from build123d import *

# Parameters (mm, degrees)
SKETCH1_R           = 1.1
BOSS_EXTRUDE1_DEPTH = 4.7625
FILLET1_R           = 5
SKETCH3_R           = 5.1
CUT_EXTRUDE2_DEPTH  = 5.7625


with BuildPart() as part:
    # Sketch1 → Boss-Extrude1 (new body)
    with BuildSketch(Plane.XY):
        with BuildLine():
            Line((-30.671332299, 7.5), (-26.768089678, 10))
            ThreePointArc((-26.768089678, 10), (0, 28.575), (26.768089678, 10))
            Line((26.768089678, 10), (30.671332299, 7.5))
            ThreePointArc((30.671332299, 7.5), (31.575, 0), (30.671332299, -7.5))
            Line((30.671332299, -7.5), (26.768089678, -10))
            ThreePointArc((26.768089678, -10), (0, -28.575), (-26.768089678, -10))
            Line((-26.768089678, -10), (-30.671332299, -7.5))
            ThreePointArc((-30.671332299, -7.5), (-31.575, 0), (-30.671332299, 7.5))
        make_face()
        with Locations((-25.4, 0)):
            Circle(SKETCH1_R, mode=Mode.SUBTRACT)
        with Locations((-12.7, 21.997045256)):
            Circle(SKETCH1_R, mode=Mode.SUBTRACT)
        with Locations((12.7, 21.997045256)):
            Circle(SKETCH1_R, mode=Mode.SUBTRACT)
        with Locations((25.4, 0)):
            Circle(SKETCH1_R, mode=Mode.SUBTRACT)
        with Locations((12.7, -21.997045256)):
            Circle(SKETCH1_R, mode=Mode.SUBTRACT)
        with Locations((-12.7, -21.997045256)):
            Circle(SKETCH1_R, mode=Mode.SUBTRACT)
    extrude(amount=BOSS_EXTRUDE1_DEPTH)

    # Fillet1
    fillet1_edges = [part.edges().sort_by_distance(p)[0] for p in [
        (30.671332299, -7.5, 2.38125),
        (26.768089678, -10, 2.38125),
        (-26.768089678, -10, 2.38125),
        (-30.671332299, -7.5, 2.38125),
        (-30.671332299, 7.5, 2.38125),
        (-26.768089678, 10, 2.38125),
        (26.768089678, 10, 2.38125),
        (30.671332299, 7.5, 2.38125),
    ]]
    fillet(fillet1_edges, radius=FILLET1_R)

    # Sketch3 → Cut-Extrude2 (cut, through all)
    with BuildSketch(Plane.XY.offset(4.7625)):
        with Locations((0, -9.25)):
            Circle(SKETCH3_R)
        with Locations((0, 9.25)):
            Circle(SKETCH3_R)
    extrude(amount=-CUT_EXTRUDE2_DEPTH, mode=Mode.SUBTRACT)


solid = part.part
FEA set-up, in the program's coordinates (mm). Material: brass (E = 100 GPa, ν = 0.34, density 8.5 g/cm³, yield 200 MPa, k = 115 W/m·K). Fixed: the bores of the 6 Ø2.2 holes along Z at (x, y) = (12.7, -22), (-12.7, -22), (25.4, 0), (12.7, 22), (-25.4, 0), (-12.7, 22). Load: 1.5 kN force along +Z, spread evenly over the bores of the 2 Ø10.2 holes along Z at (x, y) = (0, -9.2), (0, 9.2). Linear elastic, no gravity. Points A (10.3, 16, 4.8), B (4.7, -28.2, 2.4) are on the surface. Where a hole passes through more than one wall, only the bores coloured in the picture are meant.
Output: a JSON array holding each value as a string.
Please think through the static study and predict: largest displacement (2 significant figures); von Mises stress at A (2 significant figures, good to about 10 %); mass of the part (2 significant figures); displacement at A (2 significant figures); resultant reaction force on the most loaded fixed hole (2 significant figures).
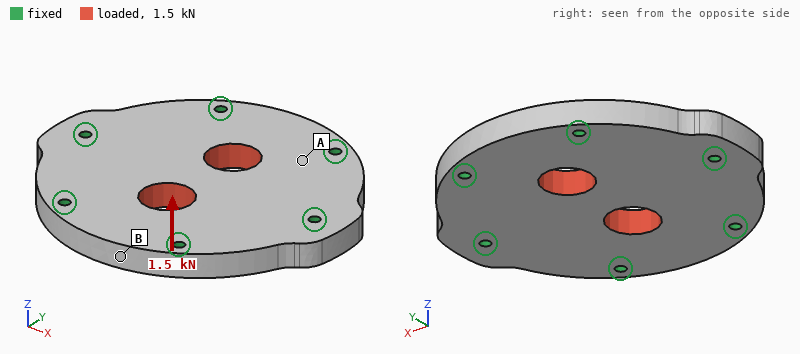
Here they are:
["26 µm", "22 MPa", "100 g", "6.7 µm", "290 N"]
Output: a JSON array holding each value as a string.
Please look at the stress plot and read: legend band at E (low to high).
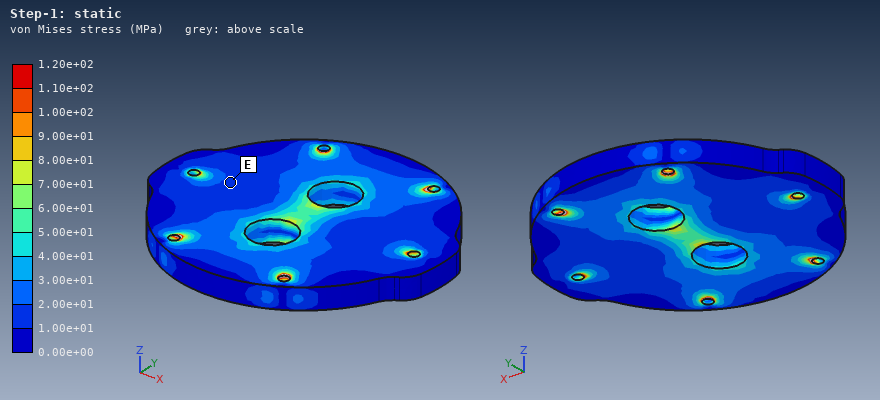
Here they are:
["1.00e+01 to 2.00e+01 MPa"]
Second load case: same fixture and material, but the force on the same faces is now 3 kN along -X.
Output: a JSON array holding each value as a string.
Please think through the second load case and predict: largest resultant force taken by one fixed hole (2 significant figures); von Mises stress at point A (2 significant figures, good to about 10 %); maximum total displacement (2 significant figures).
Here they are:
["670 N", "8.0 MPa", "2.6 µm"]
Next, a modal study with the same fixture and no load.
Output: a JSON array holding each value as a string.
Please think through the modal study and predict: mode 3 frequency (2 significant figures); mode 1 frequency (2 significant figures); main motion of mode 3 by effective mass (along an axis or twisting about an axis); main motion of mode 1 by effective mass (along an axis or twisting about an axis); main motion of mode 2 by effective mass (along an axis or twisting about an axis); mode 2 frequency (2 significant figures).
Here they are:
["17 kHz", "8900 Hz", "twisting about X", "along Z", "twisting about Y", "16 kHz"]
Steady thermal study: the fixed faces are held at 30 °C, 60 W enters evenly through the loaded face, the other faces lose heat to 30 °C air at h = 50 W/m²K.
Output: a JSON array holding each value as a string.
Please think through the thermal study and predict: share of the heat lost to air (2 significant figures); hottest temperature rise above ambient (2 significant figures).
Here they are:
["4.1 %", "28 K"]
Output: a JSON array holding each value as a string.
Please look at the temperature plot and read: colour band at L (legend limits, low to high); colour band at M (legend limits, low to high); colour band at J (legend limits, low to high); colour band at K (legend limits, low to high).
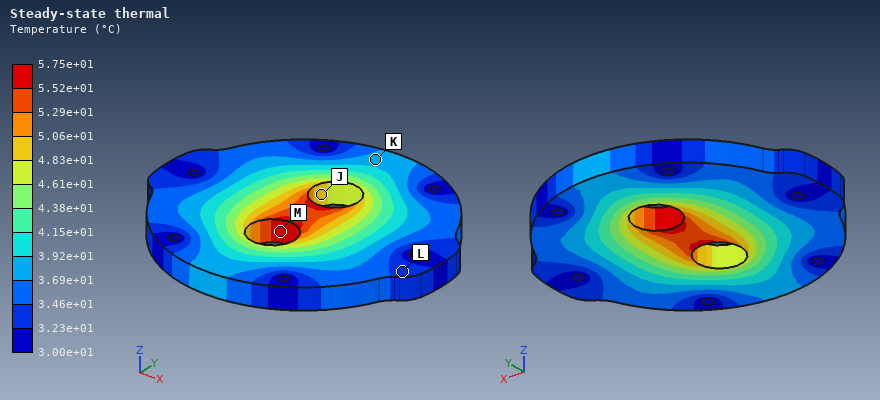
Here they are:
["3.23e+01 to 3.46e+01 °C", "5.52e+01 to 5.75e+01 °C", "4.83e+01 to 5.06e+01 °C", "3.69e+01 to 3.92e+01 °C"]
